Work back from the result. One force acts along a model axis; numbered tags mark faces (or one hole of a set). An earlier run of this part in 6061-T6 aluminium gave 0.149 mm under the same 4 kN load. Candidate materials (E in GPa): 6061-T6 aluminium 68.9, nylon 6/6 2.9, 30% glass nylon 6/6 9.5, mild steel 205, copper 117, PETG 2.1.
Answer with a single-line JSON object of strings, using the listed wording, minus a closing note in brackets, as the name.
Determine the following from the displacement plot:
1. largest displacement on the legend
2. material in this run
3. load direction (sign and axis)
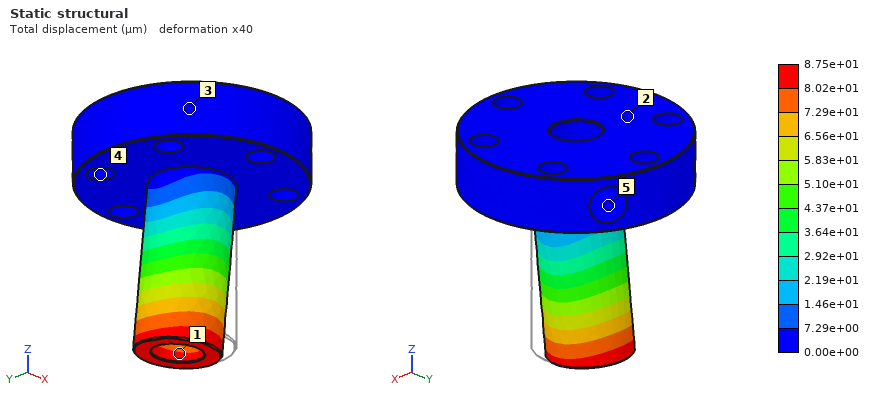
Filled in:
{"largest displacement on the legend": "8.75e+01 µm", "material in this run": "copper", "load direction": "+Y"}
